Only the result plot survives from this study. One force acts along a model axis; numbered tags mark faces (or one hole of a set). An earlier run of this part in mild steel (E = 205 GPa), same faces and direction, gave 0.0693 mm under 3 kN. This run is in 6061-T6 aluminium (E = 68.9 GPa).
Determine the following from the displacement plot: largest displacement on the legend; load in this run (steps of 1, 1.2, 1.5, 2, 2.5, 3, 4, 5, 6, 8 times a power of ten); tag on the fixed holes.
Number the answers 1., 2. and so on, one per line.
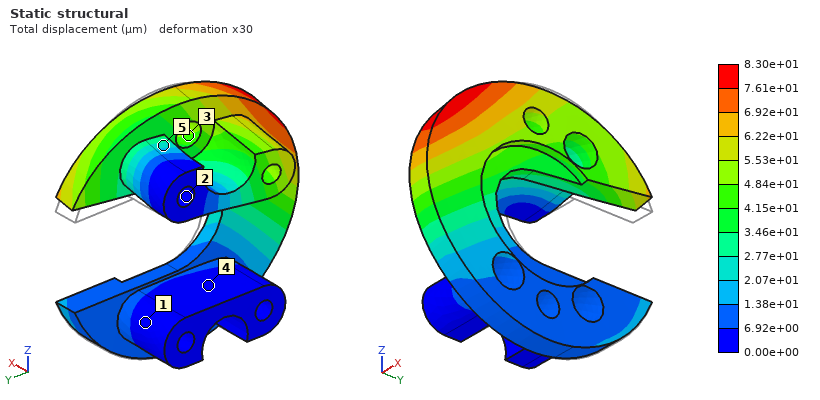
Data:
1. 8.30e+01 µm
2. 1.2 kN
3. 2
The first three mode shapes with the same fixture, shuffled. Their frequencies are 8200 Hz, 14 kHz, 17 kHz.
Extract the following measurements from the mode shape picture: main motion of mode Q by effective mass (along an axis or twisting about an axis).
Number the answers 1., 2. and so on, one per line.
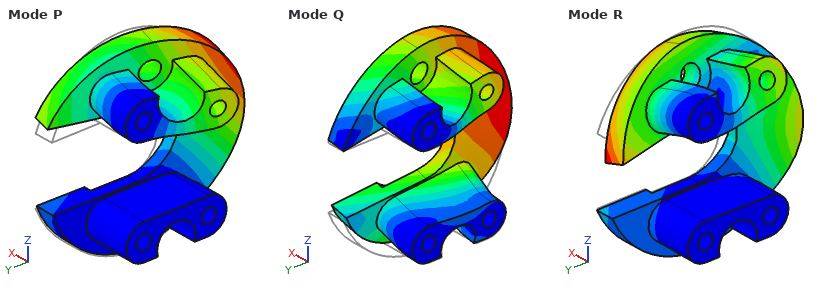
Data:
1. along Z
